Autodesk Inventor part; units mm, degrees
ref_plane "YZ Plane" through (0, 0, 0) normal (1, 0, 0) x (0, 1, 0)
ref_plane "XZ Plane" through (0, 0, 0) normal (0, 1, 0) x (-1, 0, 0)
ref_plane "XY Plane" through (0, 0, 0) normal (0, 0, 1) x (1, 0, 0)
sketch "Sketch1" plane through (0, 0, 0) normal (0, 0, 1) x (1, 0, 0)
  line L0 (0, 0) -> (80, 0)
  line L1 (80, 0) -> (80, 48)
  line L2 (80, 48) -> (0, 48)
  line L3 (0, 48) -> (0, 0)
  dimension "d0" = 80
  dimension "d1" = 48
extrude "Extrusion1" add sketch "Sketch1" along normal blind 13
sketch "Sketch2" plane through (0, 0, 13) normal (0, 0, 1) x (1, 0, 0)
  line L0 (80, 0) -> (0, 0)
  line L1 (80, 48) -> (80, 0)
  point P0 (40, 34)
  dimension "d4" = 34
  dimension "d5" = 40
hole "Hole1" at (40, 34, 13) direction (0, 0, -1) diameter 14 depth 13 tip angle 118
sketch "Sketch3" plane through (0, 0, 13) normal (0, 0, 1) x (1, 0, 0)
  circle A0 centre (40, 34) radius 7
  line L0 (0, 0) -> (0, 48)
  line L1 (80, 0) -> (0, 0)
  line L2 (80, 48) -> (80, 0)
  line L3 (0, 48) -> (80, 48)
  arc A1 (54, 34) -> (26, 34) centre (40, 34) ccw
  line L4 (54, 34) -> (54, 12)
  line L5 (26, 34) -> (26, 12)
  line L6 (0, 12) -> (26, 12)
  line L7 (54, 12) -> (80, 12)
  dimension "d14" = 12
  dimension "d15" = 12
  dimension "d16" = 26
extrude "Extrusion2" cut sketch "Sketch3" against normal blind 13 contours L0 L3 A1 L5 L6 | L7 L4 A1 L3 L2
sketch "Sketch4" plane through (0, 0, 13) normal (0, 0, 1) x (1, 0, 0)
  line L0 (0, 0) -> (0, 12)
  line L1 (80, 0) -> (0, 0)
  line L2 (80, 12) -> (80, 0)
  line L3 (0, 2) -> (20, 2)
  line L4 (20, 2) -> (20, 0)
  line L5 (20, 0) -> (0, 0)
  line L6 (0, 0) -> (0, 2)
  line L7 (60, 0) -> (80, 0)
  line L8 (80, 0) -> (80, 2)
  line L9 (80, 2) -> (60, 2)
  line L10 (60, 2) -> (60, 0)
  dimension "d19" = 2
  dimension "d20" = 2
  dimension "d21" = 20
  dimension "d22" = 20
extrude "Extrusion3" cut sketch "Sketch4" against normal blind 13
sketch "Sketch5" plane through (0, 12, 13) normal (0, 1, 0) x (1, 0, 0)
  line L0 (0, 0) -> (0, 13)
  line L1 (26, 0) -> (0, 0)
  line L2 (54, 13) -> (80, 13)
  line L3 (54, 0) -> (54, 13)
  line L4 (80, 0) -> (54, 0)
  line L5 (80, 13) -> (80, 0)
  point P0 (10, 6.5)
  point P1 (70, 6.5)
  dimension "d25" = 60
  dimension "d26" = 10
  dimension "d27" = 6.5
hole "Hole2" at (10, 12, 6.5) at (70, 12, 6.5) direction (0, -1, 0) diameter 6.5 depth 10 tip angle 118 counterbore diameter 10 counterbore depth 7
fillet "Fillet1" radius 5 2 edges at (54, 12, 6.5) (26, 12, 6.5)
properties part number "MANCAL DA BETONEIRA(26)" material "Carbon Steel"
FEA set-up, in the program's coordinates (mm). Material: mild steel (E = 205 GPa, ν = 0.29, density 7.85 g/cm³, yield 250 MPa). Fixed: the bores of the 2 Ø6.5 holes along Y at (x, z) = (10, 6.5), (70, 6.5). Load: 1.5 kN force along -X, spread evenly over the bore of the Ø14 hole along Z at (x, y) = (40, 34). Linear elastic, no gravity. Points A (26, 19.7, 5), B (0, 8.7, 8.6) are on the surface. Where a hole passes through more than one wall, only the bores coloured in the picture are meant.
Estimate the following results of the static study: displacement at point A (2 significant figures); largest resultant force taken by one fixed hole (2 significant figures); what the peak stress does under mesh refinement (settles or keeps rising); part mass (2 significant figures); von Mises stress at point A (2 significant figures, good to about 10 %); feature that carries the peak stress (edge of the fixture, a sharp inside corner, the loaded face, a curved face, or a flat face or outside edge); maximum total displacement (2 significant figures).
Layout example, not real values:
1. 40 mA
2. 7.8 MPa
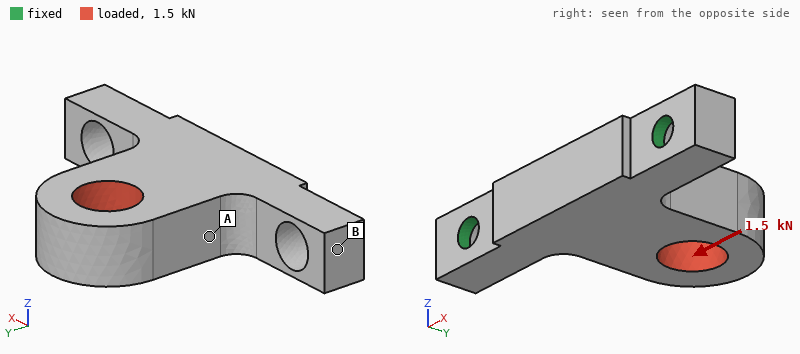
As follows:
1. 4.0 µm
2. 1.1 kN
3. keeps rising
4. 160 g
5. 18 MPa
6. edge of the fixture
7. 12 µm
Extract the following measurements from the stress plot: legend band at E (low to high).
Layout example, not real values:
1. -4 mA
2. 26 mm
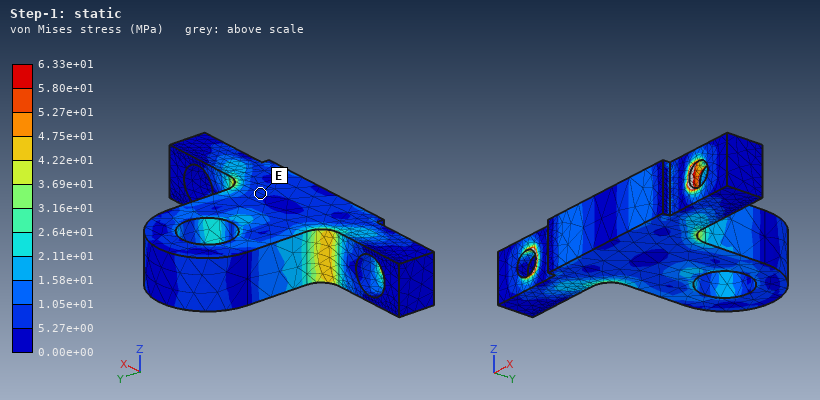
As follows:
1. 5.27e+00 to 1.05e+01 MPa
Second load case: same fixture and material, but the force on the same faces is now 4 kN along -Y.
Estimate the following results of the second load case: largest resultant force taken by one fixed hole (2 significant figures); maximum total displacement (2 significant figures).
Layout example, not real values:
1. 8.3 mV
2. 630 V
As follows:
1. 2.7 kN
2. 13 µm
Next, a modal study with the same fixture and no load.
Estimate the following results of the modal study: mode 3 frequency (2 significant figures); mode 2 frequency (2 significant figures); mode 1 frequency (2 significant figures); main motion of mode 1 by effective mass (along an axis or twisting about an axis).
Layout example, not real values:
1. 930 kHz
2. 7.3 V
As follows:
1. 8800 Hz
2. 8500 Hz
3. 2400 Hz
4. along Z
